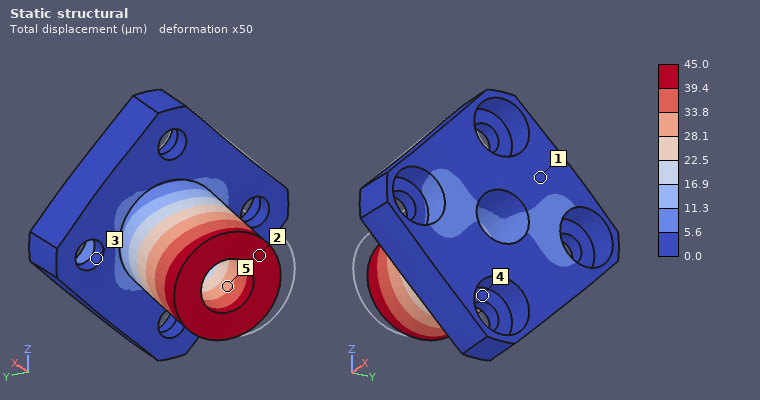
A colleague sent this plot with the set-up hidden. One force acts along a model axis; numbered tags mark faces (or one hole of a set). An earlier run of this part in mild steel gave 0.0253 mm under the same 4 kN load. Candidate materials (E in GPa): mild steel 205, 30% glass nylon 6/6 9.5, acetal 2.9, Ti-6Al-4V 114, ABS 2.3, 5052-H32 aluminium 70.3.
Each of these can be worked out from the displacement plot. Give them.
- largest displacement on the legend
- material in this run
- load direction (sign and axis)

45.0 µm
Ti-6Al-4V
+Y
